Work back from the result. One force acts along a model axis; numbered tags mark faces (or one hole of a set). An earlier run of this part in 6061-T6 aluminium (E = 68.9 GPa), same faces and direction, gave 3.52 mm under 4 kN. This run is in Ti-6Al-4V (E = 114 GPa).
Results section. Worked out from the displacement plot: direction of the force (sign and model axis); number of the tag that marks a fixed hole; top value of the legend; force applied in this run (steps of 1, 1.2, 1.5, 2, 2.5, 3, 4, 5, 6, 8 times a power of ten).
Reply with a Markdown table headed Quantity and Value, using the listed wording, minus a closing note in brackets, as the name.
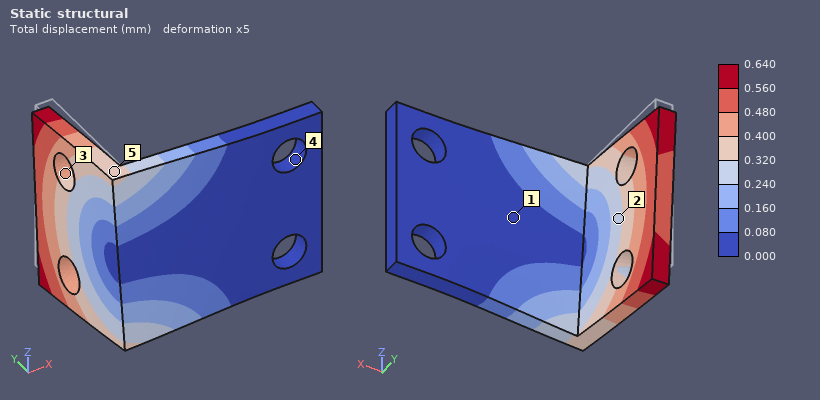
| Quantity | Value |
|---|---|
| direction of the force | -Z |
| number of the tag that marks a fixed hole | 4 |
| top value of the legend | 0.640 mm |
| force applied in this run | 1.2 kN |
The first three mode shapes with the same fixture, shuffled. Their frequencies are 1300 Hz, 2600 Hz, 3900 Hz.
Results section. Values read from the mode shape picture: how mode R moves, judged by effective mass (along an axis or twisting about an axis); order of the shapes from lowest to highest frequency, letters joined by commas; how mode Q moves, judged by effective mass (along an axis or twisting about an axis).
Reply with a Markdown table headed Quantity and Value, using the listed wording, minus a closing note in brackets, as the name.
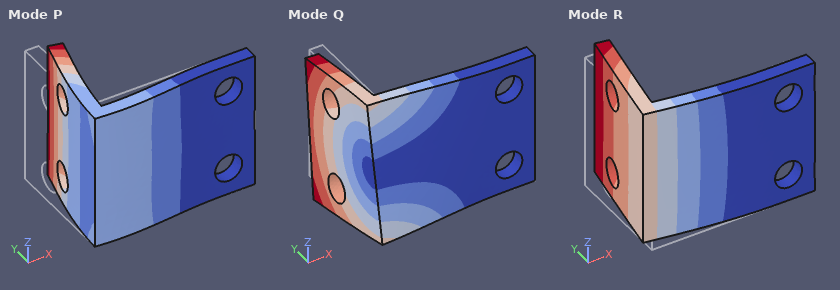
| Quantity | Value |
|---|---|
| how mode R moves, judged by effective mass | along Y |
| order of the shapes from lowest to highest frequency, letters joined by commas | R, Q, P |
| how mode Q moves, judged by effective mass | along Z |
